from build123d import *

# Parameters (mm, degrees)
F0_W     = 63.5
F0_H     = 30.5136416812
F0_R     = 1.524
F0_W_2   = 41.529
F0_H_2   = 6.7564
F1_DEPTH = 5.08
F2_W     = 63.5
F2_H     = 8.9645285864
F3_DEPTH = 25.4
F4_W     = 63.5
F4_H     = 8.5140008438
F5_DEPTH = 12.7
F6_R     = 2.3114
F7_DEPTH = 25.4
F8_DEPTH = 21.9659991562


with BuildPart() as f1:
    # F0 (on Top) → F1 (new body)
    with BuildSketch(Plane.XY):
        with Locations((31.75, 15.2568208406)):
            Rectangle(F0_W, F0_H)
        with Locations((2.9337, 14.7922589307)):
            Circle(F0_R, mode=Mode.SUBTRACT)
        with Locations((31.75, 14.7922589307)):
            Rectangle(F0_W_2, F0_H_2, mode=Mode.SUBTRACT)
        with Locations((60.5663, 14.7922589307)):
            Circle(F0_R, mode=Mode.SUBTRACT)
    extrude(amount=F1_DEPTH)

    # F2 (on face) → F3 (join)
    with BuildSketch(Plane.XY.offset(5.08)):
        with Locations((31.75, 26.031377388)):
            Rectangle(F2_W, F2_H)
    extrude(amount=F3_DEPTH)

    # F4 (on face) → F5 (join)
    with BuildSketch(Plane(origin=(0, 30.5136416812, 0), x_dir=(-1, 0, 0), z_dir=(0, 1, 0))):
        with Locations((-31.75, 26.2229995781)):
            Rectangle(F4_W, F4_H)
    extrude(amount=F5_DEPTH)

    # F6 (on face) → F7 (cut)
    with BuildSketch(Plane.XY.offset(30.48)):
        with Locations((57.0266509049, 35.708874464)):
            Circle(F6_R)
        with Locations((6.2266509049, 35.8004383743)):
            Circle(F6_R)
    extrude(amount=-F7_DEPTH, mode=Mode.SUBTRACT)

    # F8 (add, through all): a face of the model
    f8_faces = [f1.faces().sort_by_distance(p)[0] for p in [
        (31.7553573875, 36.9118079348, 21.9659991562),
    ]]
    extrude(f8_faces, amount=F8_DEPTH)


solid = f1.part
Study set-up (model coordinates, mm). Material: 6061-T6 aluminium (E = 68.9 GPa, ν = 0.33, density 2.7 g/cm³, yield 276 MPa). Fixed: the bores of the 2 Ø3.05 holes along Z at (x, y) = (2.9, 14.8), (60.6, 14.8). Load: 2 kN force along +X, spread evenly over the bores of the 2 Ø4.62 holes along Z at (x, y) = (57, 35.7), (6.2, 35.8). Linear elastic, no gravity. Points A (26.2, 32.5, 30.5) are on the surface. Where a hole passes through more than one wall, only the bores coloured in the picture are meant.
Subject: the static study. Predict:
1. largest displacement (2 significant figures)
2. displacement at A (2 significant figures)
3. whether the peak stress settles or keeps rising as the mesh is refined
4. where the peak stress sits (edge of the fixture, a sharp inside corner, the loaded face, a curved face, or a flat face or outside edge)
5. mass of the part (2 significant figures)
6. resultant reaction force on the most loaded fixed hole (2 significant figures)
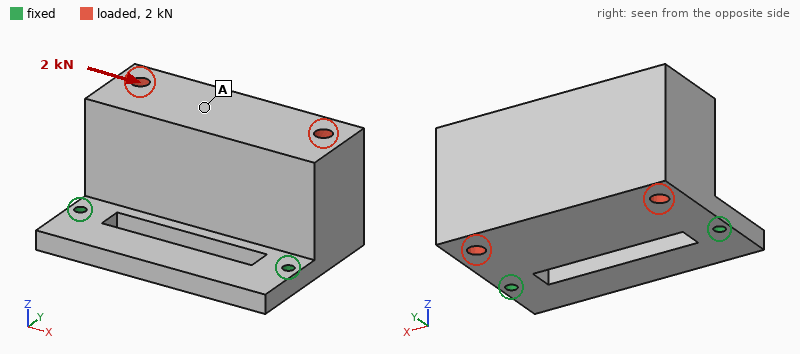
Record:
18 µm
16 µm
keeps rising
edge of the fixture
130 g
1.3 kN
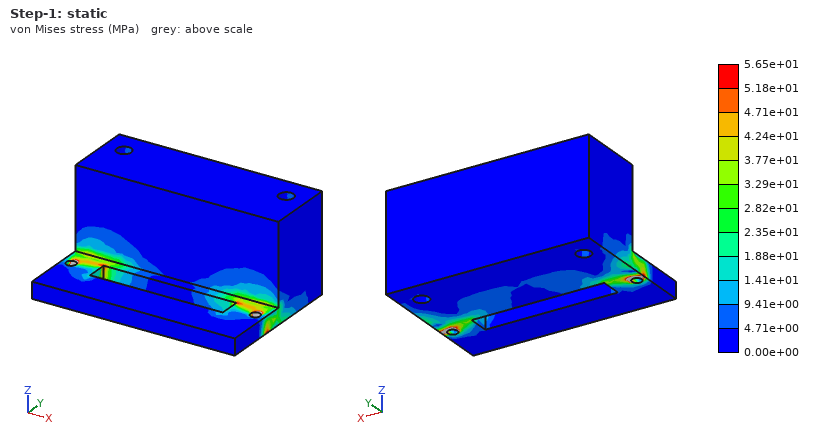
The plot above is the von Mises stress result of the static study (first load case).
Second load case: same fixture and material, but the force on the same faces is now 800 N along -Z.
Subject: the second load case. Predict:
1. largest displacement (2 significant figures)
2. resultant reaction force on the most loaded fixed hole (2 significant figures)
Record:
0.26 mm
400 N
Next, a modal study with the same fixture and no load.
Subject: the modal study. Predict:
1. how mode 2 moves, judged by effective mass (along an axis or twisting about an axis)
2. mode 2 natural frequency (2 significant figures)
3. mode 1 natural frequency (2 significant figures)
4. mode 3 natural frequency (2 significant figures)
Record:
along X
5200 Hz
970 Hz
6100 Hz
